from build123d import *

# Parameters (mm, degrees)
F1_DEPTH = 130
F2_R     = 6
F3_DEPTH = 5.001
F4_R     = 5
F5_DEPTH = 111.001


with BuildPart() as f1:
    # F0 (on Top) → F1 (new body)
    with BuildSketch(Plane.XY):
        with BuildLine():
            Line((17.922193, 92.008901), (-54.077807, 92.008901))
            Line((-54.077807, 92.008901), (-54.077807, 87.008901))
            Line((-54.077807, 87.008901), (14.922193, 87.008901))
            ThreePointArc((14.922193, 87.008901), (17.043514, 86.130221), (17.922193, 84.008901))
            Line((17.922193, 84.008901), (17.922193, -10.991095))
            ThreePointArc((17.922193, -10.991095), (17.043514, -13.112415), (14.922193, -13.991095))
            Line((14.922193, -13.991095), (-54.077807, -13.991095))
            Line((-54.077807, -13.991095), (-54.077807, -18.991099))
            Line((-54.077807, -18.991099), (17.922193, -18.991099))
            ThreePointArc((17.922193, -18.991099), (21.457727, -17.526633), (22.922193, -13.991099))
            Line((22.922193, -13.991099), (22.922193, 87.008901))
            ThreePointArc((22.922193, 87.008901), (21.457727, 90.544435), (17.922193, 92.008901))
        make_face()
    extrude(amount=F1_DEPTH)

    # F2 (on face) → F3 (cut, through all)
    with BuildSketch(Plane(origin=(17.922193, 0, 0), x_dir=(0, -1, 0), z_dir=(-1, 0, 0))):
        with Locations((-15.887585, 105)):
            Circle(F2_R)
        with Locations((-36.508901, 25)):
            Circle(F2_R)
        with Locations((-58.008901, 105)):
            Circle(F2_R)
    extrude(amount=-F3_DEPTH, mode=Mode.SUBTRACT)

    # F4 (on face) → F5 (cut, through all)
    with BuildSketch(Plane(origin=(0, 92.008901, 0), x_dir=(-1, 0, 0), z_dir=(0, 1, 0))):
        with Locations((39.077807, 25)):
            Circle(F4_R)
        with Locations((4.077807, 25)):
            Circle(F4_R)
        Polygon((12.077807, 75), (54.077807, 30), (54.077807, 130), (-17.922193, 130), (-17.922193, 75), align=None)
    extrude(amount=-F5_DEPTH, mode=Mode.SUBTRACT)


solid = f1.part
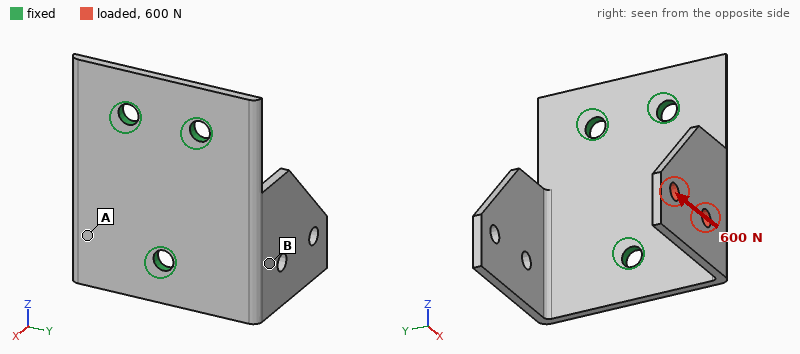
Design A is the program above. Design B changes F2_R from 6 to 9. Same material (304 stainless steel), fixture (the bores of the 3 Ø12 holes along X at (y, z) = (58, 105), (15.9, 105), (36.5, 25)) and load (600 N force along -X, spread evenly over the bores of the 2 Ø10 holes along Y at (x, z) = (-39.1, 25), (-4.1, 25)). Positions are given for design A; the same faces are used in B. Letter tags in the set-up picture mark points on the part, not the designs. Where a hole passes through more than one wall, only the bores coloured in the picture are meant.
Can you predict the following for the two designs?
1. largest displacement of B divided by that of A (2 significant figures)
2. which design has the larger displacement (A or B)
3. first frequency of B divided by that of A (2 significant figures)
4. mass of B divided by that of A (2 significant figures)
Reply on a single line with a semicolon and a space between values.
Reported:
0.87; A; 1.1; 0.98
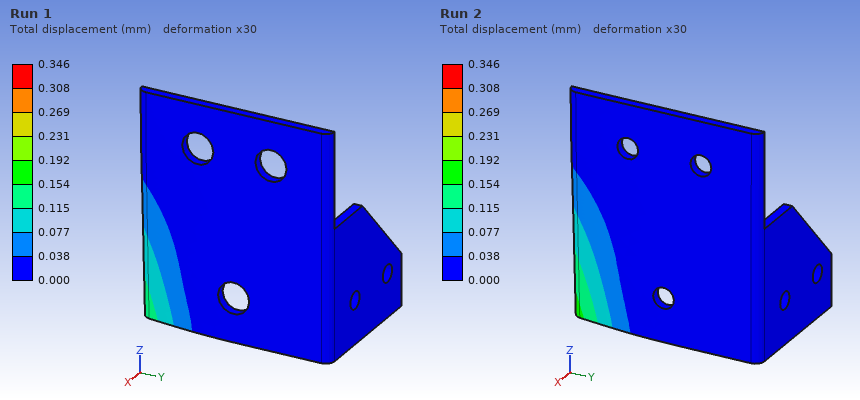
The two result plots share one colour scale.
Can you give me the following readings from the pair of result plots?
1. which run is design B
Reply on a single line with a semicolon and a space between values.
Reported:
Run 1
